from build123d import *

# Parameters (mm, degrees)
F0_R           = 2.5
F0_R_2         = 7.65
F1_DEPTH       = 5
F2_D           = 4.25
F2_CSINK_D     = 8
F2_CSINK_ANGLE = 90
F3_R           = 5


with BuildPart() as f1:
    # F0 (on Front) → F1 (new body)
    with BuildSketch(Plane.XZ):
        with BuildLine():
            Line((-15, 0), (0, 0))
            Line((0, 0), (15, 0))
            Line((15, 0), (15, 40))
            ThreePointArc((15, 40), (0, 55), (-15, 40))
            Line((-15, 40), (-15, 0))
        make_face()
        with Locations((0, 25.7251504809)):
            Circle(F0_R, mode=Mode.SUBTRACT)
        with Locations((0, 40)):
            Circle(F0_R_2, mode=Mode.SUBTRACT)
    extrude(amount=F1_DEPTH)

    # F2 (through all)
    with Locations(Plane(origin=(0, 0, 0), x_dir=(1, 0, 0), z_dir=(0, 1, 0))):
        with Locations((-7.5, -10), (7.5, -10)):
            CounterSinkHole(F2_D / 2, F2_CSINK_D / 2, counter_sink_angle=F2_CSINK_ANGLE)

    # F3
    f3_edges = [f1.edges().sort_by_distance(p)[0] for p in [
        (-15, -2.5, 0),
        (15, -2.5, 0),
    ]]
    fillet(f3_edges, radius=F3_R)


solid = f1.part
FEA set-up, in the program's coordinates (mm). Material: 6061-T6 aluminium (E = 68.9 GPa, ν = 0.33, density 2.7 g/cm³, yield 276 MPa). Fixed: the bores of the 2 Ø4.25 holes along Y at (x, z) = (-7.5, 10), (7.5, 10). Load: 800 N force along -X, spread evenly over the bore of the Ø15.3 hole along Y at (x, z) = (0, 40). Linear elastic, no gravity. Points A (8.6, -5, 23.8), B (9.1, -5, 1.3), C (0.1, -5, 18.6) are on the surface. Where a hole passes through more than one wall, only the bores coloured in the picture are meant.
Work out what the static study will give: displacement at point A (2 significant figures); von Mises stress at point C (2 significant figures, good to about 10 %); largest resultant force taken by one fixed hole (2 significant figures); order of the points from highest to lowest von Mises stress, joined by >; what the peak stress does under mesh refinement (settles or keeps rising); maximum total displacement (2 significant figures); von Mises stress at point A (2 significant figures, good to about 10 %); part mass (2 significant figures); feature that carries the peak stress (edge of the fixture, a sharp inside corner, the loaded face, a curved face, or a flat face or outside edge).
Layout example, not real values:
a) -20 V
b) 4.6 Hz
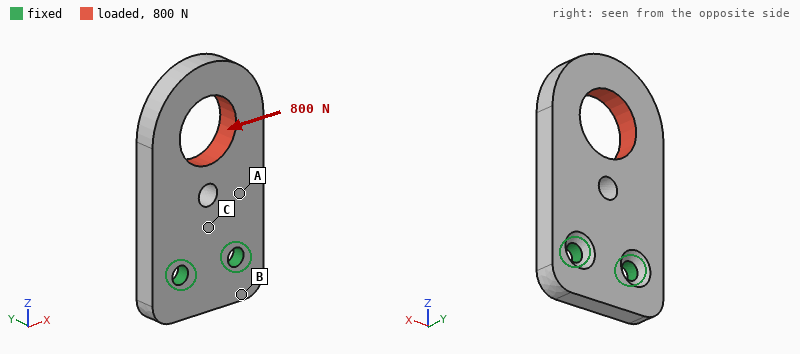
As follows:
a) 10.0 µm
b) 29 MPa
c) 1.4 kN
d) C > A > B
e) keeps rising
f) 44 µm
g) 15 MPa
h) 18 g
i) edge of the fixture
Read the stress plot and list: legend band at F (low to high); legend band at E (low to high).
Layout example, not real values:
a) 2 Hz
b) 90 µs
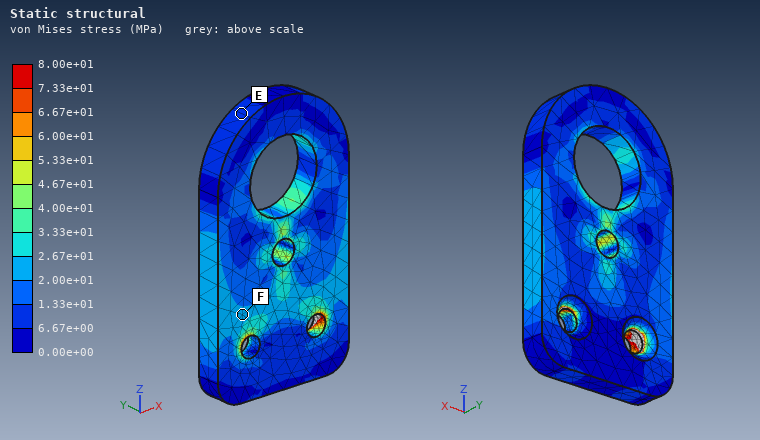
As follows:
a) 2.00e+01 to 2.67e+01 MPa
b) 6.67e+00 to 1.33e+01 MPa
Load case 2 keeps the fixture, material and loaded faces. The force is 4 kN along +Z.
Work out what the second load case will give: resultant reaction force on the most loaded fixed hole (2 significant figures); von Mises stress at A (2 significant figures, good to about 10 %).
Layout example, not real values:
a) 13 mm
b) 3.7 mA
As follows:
a) 2.0 kN
b) 30 MPa
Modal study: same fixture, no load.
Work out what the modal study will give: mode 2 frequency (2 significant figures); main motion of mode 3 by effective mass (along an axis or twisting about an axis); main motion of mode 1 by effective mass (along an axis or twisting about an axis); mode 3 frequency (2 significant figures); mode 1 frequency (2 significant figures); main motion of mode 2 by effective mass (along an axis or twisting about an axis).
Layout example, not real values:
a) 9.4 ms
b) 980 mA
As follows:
a) 6500 Hz
b) along X
c) along Y
d) 8900 Hz
e) 2300 Hz
f) twisting about Z
